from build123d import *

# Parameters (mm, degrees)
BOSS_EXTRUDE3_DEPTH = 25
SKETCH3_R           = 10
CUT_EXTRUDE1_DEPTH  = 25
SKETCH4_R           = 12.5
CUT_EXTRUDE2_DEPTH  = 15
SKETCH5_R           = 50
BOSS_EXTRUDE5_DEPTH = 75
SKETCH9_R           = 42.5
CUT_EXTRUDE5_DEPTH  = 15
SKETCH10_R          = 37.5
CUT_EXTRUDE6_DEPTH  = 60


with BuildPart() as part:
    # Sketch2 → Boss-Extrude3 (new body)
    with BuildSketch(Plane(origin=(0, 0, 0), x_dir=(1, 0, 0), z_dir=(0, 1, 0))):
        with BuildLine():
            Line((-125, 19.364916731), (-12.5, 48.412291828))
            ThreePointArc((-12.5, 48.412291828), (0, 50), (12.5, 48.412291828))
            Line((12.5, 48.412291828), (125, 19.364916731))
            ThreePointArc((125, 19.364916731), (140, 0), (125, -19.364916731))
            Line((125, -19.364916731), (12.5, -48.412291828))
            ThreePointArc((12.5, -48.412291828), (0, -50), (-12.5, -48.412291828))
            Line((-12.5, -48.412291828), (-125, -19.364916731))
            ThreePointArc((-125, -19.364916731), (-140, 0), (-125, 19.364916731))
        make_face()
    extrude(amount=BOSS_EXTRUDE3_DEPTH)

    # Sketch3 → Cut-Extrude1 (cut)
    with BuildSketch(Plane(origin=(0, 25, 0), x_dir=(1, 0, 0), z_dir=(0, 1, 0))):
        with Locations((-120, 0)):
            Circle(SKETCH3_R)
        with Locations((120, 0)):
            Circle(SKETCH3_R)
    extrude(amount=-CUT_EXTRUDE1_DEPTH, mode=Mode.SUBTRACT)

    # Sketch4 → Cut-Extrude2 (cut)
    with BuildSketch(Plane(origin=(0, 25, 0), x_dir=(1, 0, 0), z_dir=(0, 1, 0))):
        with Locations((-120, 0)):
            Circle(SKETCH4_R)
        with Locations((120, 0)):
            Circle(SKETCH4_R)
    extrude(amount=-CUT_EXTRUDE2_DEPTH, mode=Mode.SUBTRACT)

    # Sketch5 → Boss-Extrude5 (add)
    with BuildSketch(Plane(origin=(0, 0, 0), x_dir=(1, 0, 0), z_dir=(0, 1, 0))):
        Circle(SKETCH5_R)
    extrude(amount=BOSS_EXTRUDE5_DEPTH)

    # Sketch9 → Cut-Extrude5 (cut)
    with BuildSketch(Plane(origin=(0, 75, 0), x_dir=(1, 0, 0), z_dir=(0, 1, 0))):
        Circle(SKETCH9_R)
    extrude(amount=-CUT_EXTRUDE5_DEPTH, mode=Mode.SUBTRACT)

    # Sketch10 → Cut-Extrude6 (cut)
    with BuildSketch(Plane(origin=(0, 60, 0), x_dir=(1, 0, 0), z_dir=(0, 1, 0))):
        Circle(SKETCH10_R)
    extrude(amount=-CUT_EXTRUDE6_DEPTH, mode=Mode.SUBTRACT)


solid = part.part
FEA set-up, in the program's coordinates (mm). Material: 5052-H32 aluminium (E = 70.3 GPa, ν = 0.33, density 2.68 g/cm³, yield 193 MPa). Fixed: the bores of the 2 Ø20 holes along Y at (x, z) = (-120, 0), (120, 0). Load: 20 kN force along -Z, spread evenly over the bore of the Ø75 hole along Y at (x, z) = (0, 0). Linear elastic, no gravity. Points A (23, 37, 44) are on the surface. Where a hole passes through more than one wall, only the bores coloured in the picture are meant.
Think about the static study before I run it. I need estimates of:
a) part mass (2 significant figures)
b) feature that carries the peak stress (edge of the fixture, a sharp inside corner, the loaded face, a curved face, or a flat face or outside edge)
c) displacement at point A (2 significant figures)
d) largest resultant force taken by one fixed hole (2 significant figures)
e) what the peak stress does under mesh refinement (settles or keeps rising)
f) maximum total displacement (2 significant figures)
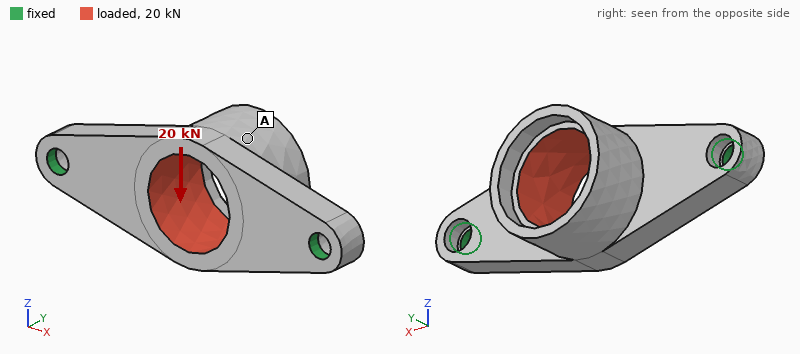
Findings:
1.3 kg
edge of the fixture
0.25 mm
10 kN
keeps rising
0.38 mm
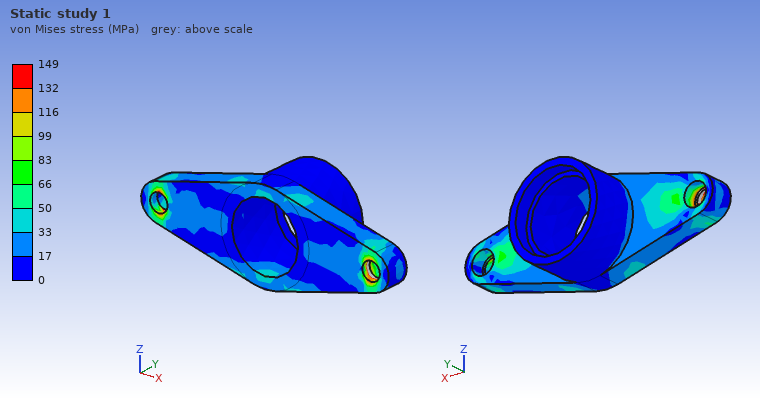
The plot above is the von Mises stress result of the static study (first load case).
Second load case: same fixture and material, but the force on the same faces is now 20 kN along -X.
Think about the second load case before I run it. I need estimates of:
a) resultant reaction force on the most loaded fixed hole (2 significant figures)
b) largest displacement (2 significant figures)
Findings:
10 kN
28 µm
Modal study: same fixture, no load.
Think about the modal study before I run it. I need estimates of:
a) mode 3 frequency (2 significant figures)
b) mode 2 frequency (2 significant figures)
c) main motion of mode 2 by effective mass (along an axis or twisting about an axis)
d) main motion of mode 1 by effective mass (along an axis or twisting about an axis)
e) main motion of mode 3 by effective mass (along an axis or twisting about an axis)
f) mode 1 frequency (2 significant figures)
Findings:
3400 Hz
1500 Hz
along Y
along Z
along Z
1300 Hz
